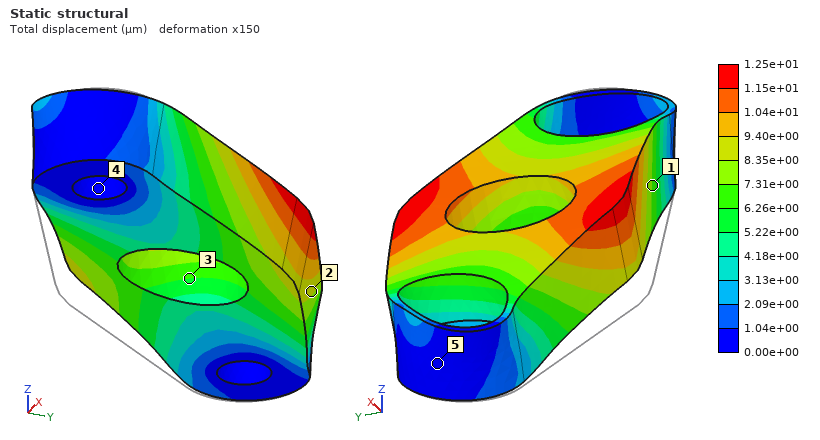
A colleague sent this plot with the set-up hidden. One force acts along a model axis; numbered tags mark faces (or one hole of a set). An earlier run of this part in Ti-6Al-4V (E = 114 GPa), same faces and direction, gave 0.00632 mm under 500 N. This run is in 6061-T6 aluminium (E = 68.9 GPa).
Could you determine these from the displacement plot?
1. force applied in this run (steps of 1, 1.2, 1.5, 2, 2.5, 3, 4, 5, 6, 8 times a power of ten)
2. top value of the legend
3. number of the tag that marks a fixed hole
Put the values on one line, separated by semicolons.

600 N; 1.25e+01 µm; 4
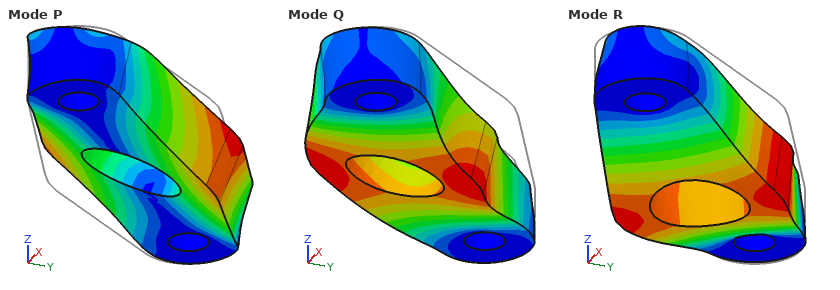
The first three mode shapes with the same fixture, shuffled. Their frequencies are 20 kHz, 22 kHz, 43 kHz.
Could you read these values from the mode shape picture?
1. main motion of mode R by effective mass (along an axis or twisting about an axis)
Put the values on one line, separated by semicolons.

along Z
